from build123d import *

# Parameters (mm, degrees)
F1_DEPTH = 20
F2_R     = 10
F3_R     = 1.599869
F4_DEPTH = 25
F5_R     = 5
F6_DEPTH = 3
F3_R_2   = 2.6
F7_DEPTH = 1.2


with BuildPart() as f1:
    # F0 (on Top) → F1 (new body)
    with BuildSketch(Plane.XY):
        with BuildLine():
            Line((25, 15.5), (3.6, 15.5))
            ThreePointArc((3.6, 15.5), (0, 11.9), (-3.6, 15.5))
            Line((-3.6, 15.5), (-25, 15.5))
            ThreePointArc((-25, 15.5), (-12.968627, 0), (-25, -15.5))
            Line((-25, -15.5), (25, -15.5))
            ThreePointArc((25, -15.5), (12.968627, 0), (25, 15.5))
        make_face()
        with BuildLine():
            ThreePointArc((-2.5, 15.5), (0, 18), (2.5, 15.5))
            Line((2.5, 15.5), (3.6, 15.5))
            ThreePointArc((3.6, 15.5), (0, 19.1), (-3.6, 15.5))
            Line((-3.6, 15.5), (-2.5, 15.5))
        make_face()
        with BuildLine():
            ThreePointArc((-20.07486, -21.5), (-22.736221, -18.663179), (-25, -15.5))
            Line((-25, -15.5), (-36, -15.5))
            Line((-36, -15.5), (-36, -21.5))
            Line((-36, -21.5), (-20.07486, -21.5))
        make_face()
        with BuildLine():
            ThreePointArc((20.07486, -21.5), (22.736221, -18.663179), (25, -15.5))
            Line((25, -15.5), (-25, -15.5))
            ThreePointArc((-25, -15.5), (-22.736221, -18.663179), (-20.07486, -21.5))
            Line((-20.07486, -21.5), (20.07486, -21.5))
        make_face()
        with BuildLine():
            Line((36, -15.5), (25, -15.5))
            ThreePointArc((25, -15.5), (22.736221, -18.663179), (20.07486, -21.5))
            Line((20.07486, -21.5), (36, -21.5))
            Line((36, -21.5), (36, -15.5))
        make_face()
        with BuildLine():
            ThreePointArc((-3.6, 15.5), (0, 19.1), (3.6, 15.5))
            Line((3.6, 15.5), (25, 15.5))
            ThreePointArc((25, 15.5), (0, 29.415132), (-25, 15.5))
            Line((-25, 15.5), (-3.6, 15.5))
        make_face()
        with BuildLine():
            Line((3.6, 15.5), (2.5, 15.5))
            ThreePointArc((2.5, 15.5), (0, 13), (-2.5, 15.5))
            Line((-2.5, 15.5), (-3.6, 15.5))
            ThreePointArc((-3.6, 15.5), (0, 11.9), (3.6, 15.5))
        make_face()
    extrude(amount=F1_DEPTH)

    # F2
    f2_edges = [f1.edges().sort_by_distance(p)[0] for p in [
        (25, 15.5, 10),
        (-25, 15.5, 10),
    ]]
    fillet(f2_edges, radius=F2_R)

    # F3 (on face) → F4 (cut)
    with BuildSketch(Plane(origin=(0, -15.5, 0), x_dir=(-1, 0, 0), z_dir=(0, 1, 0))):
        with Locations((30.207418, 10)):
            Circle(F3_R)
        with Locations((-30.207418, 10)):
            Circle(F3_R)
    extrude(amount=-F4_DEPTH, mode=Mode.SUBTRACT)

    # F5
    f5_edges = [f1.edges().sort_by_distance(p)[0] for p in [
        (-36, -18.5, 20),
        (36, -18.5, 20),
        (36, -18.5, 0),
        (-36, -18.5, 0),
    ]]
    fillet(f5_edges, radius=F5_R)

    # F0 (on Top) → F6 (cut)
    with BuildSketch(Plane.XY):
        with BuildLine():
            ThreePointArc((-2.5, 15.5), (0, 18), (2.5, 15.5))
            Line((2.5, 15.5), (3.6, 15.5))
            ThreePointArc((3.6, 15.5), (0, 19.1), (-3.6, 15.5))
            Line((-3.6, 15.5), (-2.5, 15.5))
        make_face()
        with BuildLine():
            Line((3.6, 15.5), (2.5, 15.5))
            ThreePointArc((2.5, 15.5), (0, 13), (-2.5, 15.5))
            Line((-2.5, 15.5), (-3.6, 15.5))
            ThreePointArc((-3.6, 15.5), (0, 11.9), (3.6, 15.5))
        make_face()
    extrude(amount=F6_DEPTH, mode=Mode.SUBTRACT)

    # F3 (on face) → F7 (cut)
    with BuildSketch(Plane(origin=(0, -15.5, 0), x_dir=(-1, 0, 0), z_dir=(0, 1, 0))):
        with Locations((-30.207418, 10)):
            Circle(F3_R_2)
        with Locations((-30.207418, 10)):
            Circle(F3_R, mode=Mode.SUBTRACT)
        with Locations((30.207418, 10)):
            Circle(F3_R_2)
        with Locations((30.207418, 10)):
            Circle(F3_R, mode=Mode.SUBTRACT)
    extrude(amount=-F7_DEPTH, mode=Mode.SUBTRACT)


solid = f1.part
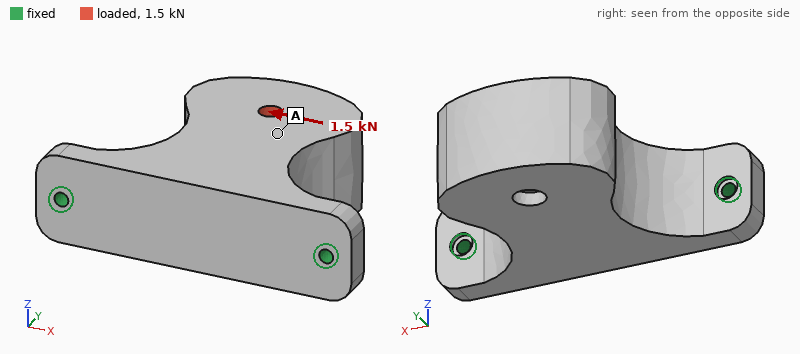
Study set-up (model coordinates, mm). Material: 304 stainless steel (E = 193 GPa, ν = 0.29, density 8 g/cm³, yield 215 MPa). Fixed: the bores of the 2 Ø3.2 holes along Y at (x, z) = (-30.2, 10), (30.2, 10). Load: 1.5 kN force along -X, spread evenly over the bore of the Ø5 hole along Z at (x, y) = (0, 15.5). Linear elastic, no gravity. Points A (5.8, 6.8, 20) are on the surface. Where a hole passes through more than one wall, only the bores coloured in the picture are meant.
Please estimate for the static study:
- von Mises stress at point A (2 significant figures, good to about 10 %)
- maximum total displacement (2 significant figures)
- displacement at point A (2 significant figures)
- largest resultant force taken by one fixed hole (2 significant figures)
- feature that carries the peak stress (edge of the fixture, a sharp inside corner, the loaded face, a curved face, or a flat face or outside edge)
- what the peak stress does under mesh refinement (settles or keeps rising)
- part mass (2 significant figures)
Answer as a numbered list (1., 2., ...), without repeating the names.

1. 8.4 MPa
2. 14 µm
3. 7.1 µm
4. 1.2 kN
5. edge of the fixture
6. keeps rising
7. 290 g
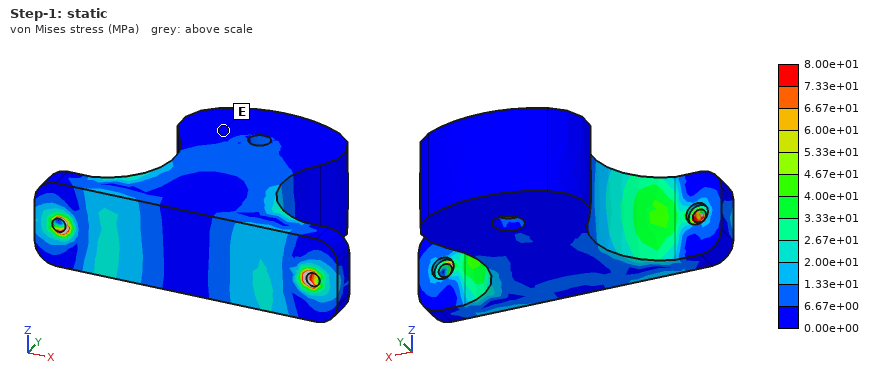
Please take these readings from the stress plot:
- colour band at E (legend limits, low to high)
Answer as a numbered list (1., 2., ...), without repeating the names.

1. 0.00e+00 to 6.67e+00 MPa
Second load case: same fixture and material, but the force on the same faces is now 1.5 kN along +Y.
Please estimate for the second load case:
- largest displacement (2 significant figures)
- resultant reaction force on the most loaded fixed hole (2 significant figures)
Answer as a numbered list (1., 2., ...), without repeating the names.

1. 12 µm
2. 1.0 kN
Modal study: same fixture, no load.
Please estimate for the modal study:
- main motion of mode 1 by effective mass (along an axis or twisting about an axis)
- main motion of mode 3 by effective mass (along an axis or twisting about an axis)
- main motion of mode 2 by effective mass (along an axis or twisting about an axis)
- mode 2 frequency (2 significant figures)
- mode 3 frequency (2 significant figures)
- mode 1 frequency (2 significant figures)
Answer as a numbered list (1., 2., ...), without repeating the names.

1. along Z
2. along Y
3. along X
4. 4800 Hz
5. 5400 Hz
6. 1300 Hz
